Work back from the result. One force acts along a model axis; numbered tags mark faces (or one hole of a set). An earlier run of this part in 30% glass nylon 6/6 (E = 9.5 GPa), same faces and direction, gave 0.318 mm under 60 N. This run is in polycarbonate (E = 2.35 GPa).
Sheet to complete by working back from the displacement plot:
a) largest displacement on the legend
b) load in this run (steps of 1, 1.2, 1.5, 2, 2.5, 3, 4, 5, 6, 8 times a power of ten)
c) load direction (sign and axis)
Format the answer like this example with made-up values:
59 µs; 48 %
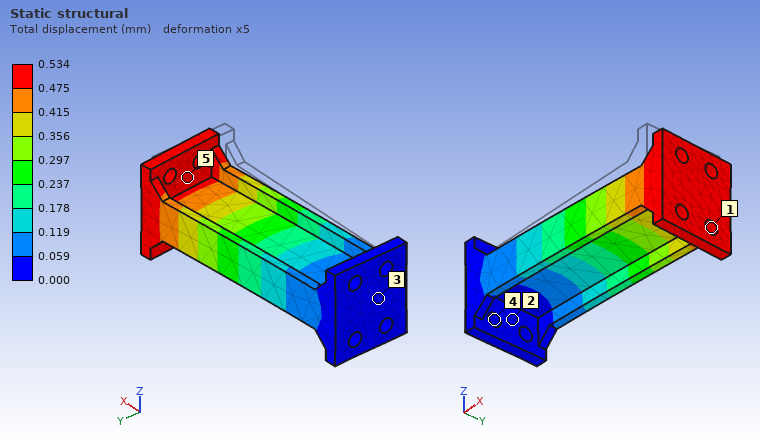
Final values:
0.534 mm; 25 N; +Y
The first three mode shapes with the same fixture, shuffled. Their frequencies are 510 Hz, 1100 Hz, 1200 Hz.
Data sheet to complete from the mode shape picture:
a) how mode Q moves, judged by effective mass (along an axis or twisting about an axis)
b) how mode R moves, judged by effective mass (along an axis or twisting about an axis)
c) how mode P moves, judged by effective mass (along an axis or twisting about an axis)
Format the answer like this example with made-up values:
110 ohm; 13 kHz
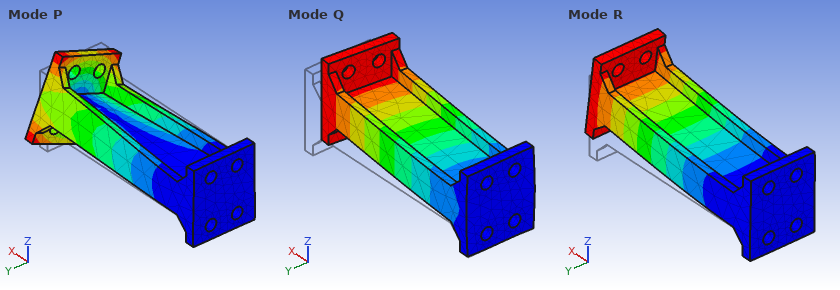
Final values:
along Y; along Z; twisting about X
